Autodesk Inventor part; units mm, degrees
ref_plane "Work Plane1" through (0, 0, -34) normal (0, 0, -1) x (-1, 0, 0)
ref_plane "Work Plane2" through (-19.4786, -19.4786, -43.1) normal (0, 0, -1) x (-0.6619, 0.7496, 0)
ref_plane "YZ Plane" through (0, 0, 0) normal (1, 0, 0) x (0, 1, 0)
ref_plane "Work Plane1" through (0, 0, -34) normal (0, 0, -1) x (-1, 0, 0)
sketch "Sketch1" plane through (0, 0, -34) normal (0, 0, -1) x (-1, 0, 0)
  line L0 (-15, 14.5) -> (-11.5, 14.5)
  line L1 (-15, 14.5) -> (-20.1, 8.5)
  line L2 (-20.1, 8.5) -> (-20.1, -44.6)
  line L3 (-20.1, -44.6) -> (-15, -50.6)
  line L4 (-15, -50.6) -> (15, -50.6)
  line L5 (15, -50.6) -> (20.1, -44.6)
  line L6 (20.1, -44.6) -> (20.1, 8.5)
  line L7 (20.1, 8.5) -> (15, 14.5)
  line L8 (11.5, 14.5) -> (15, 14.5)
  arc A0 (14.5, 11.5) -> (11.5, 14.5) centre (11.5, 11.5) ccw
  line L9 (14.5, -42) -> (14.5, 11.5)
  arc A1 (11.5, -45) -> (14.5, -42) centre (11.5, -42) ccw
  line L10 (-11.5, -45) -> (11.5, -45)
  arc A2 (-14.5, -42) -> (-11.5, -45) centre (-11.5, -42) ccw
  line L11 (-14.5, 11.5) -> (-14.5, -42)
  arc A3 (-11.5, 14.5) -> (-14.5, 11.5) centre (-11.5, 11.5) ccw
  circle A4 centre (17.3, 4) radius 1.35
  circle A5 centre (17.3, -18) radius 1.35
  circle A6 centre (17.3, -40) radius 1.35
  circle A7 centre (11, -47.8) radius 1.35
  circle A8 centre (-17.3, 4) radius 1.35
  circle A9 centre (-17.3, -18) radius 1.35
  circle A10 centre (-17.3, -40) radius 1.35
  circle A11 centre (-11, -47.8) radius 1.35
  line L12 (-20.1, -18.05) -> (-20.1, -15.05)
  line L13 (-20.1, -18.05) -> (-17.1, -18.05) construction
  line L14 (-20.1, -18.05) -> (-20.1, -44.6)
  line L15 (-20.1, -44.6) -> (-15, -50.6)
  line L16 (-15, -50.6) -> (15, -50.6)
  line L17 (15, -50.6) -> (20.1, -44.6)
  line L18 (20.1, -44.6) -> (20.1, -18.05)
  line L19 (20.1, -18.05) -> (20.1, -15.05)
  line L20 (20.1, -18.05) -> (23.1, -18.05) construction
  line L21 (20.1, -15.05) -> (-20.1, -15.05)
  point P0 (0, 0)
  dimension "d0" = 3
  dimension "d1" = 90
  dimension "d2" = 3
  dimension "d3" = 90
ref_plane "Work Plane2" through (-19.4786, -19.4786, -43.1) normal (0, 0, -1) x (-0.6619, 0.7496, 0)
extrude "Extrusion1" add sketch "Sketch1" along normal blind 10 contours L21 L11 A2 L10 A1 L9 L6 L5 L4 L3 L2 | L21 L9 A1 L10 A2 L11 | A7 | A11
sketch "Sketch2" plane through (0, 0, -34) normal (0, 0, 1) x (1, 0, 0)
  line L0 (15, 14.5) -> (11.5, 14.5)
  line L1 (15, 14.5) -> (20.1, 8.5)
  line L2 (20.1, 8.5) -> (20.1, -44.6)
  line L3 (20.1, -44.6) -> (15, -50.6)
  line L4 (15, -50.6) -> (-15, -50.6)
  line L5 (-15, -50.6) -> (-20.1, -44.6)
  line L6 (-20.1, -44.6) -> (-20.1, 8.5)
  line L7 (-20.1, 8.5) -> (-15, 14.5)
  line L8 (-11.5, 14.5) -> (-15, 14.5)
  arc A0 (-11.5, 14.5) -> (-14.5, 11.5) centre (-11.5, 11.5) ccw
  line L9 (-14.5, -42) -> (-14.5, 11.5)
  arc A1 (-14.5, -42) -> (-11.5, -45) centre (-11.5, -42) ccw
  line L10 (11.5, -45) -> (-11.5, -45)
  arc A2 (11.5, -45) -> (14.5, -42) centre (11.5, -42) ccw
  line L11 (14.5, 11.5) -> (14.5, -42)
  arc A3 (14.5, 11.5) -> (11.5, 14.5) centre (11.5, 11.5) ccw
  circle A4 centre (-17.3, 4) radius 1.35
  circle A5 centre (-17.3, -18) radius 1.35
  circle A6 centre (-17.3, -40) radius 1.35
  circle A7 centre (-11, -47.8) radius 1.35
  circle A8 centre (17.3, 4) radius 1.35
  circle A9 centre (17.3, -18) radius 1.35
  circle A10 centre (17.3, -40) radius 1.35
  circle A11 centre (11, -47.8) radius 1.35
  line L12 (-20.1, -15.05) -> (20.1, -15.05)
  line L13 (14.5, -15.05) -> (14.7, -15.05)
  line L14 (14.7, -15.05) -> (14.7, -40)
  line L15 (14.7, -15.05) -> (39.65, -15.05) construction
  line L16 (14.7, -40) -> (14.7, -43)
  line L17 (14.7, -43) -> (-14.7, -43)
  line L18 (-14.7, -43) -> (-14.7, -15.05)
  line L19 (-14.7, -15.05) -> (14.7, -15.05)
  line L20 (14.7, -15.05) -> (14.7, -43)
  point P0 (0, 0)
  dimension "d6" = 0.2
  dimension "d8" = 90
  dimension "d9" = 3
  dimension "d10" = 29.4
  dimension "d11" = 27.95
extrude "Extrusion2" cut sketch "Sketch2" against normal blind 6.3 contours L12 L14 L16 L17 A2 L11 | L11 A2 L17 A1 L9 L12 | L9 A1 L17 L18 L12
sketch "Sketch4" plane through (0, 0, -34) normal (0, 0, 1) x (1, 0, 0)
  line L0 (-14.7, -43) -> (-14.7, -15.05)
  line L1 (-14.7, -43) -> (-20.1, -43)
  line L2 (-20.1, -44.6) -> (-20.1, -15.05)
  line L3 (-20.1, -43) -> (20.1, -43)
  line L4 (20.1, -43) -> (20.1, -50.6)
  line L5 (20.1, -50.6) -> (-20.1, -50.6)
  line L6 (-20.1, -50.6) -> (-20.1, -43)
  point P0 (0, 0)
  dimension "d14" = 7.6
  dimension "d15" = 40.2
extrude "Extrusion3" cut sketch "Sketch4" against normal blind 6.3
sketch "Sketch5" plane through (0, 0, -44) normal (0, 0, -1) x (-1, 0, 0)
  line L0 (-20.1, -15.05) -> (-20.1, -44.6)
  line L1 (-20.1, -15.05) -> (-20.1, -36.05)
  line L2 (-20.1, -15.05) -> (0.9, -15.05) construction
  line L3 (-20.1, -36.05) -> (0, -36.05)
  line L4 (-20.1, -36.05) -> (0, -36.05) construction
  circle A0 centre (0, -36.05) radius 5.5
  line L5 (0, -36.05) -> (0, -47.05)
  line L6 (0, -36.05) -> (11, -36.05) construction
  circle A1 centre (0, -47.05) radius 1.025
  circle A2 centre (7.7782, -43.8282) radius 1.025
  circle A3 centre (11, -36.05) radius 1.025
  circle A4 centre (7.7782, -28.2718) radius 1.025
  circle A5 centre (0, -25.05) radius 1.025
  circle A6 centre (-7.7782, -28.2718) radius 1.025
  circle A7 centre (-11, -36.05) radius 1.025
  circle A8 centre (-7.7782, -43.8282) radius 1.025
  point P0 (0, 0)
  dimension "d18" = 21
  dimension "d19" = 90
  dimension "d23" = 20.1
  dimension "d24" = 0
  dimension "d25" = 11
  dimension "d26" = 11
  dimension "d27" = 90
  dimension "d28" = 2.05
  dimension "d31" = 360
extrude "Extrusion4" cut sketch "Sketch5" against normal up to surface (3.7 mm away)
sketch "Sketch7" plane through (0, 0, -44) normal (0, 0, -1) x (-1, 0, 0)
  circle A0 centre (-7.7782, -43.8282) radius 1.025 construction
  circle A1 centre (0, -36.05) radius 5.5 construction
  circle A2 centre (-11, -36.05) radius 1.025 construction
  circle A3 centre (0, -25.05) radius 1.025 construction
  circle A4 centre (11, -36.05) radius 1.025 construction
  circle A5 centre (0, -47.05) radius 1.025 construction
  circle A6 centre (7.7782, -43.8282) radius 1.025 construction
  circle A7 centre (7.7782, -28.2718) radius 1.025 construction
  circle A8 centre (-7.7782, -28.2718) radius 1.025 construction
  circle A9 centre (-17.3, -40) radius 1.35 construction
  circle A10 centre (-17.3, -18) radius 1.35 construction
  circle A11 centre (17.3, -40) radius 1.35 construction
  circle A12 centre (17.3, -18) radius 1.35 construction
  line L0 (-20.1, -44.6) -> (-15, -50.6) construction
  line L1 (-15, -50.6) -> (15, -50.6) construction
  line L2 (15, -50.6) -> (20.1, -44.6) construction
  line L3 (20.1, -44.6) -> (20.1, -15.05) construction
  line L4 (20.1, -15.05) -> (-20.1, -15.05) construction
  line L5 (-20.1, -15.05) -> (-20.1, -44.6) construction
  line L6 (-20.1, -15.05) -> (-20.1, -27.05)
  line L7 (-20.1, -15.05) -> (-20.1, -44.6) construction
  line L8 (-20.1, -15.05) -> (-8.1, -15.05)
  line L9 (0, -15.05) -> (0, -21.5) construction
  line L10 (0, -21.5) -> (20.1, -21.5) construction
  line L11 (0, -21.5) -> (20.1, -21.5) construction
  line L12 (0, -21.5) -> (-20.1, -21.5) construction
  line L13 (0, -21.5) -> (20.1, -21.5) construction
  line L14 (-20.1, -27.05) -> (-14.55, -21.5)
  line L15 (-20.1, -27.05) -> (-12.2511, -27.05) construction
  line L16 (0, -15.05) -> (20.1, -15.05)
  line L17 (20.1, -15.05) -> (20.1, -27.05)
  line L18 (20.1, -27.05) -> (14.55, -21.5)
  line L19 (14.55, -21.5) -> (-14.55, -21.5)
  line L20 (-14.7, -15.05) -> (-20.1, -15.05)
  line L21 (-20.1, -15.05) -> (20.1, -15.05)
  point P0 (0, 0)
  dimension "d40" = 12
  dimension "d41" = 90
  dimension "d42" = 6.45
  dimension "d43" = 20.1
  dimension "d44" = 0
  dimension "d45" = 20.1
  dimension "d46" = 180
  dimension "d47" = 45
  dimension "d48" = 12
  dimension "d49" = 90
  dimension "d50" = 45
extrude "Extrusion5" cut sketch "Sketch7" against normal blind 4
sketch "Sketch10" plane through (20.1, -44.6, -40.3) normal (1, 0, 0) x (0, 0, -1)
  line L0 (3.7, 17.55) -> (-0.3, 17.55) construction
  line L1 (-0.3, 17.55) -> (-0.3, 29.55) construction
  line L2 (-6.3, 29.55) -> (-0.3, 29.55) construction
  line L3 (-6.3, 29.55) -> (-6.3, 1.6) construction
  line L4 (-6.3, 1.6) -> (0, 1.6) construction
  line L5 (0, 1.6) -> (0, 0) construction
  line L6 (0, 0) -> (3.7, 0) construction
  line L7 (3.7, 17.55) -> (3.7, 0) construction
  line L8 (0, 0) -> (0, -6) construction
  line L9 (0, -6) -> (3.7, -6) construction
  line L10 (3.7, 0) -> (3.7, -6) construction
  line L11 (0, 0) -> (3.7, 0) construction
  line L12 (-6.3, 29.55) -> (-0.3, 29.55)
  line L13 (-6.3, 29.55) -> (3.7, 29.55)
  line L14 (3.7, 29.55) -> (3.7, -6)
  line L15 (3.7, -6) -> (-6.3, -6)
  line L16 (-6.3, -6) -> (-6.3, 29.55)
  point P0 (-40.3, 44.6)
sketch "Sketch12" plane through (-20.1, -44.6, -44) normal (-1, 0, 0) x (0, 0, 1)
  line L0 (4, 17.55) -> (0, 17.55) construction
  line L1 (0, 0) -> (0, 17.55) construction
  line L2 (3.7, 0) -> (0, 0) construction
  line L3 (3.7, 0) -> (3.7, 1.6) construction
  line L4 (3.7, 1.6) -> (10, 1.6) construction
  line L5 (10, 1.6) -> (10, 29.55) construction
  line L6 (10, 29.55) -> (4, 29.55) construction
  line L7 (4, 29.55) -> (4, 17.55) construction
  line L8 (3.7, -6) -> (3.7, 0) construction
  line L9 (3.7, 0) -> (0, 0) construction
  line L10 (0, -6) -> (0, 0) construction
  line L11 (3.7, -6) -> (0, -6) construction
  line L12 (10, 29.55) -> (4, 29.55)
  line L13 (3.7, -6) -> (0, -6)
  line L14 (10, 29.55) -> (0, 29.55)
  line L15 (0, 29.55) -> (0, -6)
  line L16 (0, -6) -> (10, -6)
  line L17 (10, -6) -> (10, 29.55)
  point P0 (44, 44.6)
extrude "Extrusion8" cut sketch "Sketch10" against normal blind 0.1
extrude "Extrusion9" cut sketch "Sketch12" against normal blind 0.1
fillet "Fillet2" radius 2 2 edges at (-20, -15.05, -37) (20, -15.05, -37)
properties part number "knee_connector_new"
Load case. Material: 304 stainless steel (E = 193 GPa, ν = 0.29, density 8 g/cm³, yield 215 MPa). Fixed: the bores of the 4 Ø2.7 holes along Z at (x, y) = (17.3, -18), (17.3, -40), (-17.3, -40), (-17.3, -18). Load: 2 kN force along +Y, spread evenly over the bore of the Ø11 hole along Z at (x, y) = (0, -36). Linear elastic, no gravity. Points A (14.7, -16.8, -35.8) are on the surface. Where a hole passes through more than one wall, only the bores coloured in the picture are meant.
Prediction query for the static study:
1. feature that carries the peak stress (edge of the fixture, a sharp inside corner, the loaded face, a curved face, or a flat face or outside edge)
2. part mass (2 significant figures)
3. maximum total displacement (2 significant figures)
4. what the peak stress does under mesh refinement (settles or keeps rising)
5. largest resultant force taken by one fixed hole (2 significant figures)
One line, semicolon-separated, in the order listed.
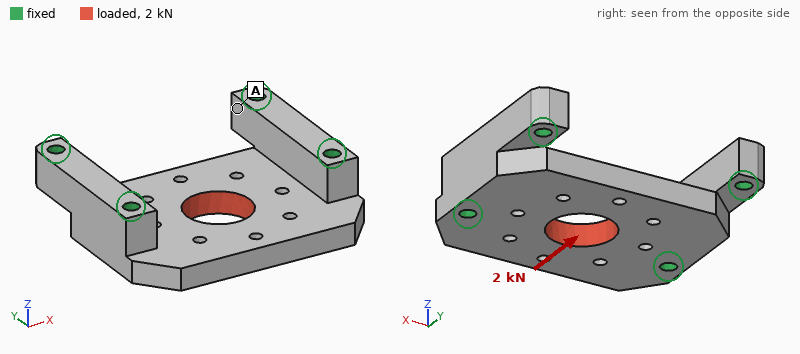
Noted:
a sharp inside corner; 42 g; 3.7 µm; keeps rising; 850 N
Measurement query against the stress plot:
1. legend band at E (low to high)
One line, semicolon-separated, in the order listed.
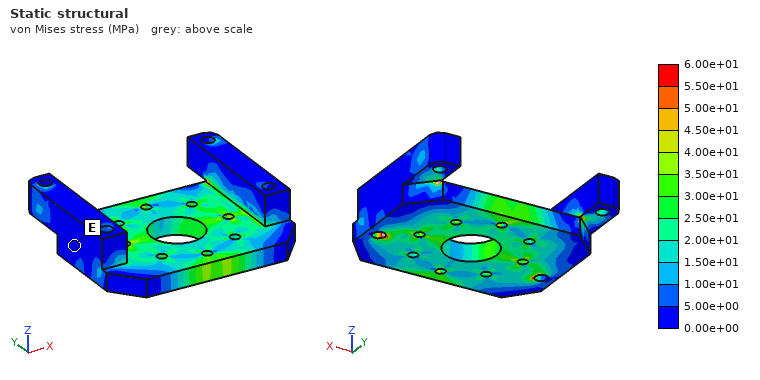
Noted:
0.00e+00 to 5.00e+00 MPa
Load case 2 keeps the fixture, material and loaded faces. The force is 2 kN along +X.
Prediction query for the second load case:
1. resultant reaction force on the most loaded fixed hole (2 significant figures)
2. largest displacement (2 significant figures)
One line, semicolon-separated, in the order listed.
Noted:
890 N; 2.5 µm
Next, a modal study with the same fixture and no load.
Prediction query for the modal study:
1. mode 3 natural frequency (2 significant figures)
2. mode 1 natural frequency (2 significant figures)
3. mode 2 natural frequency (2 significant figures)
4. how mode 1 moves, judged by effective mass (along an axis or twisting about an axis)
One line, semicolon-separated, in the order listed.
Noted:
29 kHz; 14 kHz; 15 kHz; along Z
